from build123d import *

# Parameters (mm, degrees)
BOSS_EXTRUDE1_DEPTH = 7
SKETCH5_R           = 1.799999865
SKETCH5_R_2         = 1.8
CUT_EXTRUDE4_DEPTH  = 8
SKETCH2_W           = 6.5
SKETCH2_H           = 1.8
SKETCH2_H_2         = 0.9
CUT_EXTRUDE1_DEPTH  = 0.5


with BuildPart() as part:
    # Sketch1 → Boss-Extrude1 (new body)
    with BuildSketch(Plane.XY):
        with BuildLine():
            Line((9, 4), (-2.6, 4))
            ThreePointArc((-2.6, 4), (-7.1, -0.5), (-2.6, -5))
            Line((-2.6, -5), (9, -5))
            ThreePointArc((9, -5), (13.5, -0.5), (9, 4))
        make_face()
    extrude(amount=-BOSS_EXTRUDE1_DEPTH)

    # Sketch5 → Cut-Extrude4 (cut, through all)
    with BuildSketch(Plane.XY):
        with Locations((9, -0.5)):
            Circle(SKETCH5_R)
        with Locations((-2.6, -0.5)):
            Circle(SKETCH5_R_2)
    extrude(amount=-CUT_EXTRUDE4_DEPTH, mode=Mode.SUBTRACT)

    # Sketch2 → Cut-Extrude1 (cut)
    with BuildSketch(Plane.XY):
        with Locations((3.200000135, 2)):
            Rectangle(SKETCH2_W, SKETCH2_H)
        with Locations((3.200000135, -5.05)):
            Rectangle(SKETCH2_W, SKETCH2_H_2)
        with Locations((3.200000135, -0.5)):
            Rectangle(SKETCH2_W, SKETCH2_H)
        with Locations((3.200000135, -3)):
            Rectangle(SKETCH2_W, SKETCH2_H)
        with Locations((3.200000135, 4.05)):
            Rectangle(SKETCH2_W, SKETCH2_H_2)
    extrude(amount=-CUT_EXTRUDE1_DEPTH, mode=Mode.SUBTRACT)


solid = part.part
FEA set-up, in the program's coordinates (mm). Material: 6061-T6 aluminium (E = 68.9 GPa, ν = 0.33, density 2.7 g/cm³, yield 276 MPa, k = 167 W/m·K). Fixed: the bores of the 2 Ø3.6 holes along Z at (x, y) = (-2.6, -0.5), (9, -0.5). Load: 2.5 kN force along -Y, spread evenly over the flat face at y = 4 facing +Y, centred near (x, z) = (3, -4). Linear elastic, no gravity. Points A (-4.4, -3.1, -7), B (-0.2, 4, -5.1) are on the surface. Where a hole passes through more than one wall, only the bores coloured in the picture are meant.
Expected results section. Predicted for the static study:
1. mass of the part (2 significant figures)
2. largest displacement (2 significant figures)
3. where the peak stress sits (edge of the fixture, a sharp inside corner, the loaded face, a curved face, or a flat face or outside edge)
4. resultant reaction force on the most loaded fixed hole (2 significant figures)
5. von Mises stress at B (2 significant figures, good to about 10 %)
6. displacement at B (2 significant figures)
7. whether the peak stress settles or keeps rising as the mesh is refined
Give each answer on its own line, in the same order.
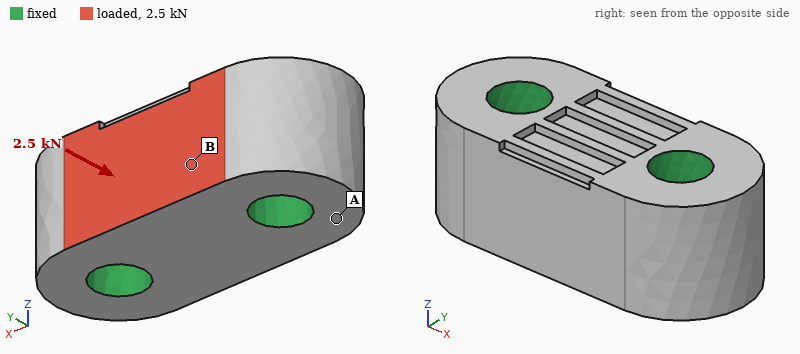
2.7 g
3.7 µm
edge of the fixture
1.3 kN
28 MPa
2.4 µm
keeps rising
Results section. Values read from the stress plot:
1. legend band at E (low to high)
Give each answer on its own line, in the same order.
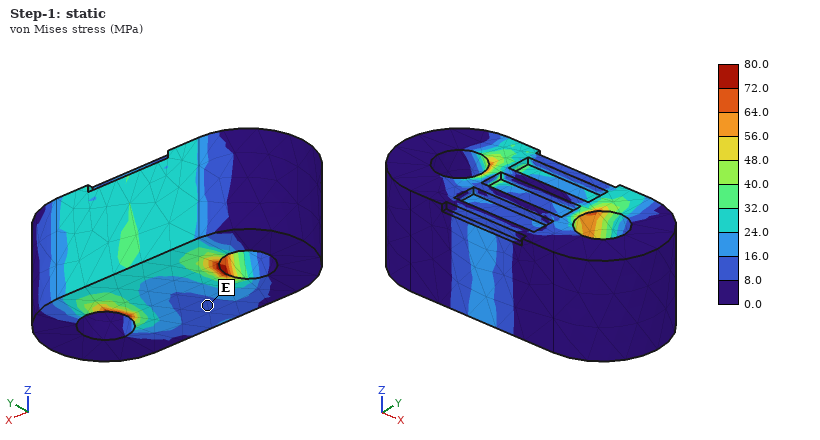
8.0 to 16.0 MPa
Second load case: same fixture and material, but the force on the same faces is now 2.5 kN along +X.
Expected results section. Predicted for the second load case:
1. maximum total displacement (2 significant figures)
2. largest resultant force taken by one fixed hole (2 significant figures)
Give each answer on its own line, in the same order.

4.0 µm
1.4 kN
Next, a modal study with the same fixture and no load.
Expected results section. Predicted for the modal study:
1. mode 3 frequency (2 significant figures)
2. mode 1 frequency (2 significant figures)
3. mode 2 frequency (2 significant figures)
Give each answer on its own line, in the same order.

140 kHz
130 kHz
130 kHz
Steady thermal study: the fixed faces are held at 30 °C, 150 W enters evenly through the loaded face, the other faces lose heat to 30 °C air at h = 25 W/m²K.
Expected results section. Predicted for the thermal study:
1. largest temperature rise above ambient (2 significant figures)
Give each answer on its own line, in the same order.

49 K
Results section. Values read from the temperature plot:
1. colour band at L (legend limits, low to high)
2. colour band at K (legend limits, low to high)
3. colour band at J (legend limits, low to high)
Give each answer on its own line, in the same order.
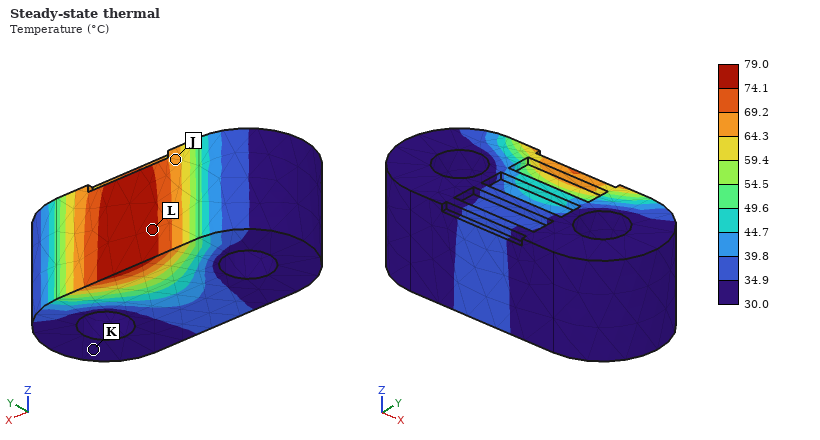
74.1 to 79.0 °C
30.0 to 34.9 °C
64.3 to 69.2 °C
